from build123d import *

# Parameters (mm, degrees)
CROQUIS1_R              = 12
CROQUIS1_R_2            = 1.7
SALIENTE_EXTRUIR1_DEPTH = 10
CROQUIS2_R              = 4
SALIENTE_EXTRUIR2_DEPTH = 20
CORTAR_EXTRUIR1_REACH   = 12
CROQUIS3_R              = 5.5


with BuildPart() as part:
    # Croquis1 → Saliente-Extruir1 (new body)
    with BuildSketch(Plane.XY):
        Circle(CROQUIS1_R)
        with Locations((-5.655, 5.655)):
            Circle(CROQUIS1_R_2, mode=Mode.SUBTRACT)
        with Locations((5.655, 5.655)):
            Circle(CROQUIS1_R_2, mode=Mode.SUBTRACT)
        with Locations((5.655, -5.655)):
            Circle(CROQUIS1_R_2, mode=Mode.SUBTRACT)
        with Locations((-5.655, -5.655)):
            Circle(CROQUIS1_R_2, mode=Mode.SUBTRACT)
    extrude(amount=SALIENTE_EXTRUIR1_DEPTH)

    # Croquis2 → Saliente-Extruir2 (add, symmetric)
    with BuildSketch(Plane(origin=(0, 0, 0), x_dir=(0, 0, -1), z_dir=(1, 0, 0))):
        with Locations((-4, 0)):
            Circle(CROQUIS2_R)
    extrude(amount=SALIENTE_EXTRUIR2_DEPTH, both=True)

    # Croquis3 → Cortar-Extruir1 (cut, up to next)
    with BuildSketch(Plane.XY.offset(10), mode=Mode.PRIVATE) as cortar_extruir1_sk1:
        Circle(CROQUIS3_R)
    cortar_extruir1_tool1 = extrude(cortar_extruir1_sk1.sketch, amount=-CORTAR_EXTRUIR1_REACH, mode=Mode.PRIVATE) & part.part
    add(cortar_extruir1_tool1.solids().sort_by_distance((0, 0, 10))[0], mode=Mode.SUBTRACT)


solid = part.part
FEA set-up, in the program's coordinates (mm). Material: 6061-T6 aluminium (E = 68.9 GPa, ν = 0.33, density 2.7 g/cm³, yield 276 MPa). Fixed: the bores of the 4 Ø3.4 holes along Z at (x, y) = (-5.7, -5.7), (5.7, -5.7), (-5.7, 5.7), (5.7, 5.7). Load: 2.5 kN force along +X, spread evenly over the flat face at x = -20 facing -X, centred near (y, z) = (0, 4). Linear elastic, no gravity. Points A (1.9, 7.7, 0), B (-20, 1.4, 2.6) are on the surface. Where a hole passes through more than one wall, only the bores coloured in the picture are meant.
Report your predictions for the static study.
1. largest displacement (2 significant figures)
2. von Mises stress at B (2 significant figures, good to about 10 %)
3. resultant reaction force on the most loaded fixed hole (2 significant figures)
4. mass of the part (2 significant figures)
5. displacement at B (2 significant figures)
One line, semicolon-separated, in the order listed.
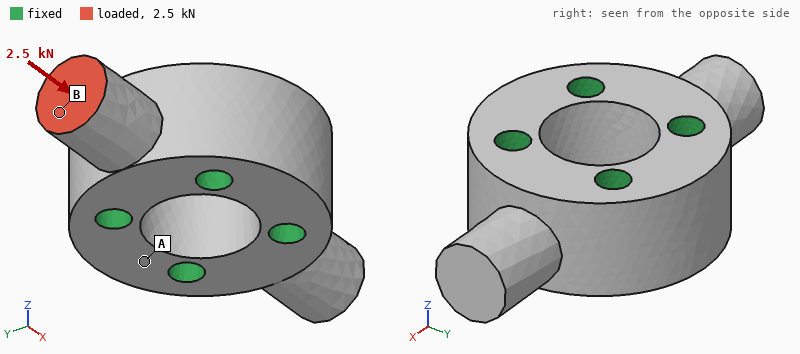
11 µm; 50 MPa; 1.4 kN; 11 g; 10 µm
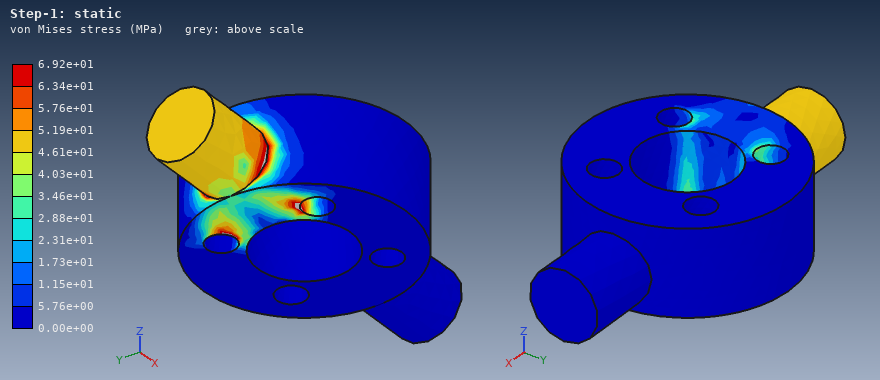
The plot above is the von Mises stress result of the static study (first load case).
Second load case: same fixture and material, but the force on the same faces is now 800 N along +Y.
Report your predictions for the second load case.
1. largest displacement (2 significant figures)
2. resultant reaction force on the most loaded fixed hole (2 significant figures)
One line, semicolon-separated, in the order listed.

30 µm; 1.0 kN
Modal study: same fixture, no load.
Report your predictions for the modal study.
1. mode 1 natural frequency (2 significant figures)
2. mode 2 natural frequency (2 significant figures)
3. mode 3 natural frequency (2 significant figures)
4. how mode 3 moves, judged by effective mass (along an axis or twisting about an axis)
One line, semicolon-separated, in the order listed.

35 kHz; 35 kHz; 43 kHz; twisting about Z
